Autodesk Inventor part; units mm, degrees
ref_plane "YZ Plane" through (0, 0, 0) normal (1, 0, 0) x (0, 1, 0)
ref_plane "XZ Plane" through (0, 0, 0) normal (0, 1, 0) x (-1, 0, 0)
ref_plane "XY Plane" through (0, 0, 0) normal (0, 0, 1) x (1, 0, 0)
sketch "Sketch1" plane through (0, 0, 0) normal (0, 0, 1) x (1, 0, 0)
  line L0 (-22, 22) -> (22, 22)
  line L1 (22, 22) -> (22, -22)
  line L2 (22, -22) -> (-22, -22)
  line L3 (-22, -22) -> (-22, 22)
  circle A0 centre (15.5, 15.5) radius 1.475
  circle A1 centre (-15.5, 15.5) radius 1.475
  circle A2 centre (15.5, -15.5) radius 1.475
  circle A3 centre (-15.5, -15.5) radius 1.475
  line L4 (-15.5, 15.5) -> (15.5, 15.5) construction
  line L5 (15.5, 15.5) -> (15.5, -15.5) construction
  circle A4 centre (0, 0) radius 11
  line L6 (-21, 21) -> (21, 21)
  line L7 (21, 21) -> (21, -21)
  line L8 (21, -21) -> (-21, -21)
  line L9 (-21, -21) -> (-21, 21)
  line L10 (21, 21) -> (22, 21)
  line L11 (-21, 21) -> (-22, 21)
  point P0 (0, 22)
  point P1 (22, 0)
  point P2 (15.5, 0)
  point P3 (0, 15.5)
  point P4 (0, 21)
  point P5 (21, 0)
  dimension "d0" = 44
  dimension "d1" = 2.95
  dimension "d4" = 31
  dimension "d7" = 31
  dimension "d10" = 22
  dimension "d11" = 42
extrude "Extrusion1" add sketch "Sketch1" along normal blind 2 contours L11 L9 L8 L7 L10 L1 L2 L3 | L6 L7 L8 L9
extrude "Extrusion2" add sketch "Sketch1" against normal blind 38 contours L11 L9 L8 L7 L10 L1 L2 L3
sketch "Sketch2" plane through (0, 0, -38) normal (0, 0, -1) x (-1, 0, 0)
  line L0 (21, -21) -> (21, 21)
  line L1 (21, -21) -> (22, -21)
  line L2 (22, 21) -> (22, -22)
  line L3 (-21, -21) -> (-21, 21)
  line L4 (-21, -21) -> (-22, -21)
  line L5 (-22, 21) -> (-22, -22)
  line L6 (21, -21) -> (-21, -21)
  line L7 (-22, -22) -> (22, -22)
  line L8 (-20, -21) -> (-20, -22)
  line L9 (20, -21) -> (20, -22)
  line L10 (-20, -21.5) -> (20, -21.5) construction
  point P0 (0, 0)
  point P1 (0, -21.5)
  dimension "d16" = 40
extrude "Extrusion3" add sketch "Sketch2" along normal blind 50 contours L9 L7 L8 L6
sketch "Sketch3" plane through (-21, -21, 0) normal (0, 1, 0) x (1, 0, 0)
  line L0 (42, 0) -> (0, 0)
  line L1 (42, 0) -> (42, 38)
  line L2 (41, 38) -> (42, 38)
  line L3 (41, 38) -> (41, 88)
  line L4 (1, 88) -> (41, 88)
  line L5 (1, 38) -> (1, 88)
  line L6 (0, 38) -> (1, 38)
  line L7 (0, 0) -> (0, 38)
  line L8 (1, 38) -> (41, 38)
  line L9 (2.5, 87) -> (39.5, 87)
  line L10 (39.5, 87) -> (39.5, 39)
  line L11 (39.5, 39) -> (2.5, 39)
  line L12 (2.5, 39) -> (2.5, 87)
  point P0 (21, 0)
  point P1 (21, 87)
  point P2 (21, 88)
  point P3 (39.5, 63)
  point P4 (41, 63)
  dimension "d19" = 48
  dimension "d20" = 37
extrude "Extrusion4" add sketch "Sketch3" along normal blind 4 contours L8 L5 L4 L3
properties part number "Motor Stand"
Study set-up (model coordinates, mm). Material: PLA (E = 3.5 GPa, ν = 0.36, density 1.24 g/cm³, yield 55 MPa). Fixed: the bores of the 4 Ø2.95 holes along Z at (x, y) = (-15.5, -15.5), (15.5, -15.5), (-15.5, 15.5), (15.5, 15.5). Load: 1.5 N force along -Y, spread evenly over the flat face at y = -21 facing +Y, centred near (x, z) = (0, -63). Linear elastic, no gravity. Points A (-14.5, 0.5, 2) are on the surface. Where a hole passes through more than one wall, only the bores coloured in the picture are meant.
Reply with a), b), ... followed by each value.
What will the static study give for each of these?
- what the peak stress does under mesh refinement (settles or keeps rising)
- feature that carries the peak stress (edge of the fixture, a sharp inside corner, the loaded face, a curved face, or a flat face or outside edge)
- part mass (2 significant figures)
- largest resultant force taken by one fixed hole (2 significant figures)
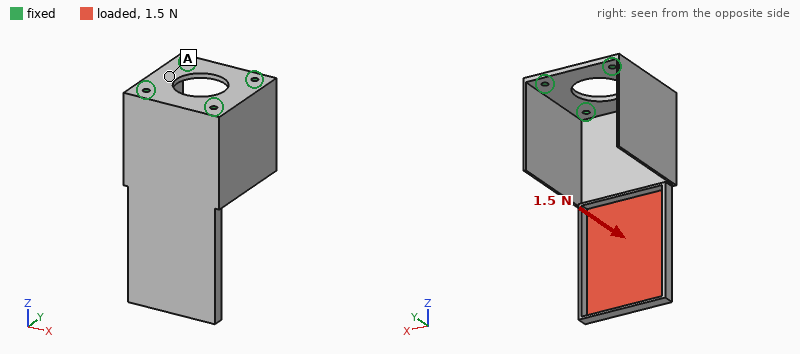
a) keeps rising
b) a sharp inside corner
c) 13 g
d) 1.5 N
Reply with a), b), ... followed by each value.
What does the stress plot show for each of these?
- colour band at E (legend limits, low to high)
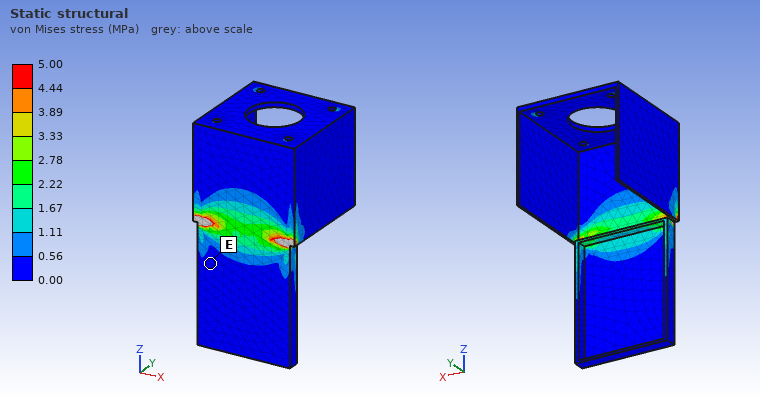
a) 0.00 to 0.56 MPa
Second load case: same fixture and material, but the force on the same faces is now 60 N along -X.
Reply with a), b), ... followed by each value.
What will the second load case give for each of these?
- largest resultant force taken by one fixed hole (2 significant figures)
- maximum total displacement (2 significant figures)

a) 130 N
b) 1.2 mm
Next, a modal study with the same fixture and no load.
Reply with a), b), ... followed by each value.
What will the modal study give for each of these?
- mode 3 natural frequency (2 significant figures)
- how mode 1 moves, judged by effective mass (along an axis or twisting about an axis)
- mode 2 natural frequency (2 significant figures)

a) 310 Hz
b) along Y
c) 300 Hz
